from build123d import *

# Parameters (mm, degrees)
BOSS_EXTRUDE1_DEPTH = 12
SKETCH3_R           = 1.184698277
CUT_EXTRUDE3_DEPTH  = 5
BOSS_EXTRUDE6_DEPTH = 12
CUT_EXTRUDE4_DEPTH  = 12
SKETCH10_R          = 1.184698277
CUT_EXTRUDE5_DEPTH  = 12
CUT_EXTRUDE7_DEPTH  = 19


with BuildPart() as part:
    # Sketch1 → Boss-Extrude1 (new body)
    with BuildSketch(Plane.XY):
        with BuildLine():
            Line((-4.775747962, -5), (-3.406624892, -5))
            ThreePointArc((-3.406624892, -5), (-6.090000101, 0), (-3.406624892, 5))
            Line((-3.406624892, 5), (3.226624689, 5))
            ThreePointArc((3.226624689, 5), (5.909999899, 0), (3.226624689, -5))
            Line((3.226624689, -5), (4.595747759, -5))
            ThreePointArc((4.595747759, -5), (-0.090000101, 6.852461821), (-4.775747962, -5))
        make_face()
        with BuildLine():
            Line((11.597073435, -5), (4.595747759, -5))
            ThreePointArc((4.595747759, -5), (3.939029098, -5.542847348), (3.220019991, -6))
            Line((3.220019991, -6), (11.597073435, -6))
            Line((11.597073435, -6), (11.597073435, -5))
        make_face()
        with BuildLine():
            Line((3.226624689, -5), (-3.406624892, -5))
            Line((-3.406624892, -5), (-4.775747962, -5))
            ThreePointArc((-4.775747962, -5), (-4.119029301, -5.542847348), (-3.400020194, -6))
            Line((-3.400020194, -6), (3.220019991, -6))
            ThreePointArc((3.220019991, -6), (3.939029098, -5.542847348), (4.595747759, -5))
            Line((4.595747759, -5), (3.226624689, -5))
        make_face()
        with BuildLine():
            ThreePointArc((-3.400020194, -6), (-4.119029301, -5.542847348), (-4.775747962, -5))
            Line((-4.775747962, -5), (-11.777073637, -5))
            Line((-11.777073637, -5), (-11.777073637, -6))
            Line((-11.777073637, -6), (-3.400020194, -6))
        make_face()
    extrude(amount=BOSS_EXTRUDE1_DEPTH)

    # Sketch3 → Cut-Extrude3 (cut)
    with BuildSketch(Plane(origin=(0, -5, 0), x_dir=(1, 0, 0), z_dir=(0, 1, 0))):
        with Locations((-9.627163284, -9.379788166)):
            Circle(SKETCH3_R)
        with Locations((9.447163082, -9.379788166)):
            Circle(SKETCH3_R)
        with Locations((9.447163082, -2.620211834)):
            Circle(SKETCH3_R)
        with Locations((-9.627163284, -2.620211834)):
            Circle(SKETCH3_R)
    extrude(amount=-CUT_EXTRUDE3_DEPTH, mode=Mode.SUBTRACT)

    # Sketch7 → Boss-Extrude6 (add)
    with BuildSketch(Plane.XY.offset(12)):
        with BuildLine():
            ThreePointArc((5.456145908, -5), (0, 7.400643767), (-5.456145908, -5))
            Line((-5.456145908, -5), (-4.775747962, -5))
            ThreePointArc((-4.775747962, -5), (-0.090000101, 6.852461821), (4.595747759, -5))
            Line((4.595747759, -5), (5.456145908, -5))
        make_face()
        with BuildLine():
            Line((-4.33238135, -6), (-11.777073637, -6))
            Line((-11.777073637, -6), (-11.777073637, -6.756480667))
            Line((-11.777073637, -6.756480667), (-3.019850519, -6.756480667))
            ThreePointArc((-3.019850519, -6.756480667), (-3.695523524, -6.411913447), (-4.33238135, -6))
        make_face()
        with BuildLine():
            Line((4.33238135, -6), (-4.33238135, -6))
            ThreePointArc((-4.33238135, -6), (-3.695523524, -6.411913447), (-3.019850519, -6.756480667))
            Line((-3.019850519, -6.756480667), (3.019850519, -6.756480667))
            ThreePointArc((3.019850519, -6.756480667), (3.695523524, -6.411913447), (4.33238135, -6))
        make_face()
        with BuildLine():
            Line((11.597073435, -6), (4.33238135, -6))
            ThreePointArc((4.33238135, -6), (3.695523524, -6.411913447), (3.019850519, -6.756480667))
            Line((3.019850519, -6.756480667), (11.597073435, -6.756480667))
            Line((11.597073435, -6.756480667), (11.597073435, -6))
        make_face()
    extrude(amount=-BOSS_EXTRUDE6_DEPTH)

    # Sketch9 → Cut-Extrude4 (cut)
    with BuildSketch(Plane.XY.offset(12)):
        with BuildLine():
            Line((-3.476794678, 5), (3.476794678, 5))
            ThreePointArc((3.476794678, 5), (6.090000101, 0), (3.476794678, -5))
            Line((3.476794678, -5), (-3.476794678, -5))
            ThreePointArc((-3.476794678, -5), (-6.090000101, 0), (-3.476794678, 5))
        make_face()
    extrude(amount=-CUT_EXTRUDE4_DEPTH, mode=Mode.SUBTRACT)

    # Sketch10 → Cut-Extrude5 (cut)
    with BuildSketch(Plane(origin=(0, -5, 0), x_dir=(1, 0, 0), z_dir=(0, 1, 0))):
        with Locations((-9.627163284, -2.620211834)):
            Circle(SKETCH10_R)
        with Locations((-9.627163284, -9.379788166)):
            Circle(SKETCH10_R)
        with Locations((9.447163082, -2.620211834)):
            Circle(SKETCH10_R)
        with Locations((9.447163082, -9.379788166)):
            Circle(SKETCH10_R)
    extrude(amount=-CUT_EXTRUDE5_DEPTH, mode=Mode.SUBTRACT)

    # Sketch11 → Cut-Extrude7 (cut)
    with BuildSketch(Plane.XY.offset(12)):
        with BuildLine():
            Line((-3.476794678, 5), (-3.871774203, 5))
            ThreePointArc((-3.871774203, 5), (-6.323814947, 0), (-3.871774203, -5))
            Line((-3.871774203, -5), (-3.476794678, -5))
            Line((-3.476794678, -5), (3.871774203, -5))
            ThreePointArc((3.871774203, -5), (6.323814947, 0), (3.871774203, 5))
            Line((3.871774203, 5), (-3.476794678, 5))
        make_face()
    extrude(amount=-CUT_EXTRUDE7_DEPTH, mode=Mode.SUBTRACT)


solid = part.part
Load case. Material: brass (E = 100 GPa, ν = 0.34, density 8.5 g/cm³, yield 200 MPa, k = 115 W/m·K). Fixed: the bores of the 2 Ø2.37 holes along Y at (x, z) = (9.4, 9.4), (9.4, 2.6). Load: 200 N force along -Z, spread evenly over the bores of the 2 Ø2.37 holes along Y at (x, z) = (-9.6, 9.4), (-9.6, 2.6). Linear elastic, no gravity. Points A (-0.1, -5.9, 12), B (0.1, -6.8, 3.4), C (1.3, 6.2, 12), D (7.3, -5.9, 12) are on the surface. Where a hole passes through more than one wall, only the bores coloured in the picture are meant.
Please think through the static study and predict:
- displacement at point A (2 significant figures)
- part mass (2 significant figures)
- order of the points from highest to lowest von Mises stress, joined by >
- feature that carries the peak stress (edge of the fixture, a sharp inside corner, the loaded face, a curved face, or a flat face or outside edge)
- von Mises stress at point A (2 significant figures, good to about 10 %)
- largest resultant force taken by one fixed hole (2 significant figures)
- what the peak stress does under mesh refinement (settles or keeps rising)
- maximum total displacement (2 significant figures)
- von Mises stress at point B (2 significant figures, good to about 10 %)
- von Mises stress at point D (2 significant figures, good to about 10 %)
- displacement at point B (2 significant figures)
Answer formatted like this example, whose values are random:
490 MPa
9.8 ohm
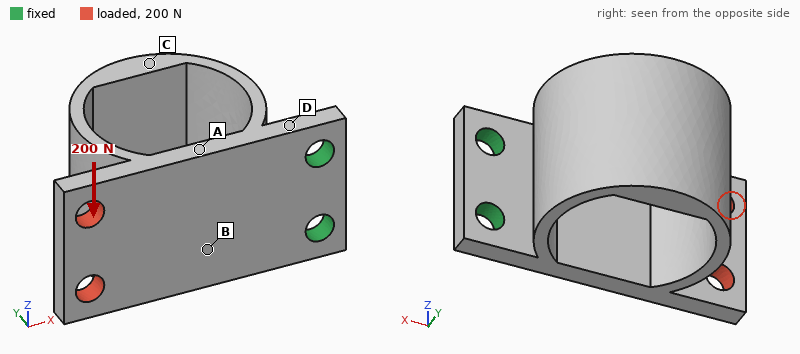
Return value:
11 µm
8.2 g
D > A > B > C
edge of the fixture
45 MPa
470 N
keeps rising
29 µm
29 MPa
60 MPa
8.4 µm
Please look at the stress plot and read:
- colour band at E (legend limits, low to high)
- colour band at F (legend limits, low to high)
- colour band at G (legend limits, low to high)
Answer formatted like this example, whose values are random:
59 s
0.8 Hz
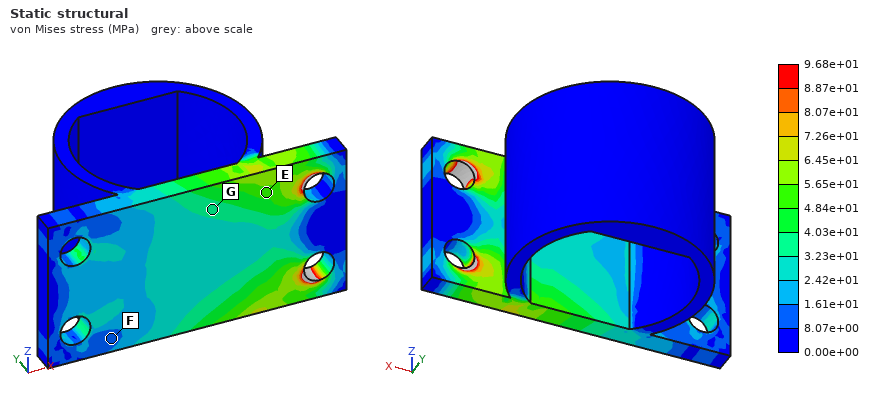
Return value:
4.84e+01 to 5.65e+01 MPa
8.07e+00 to 1.61e+01 MPa
3.23e+01 to 4.03e+01 MPa
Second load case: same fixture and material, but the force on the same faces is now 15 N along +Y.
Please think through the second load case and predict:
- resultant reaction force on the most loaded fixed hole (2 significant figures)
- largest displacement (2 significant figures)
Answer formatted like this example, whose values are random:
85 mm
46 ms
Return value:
7.6 N
54 µm
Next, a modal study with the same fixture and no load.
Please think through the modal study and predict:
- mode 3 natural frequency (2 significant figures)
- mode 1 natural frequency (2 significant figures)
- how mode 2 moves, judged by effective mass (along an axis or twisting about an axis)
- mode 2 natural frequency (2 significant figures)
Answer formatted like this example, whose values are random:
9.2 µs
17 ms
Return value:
5500 Hz
1500 Hz
along Z
4100 Hz
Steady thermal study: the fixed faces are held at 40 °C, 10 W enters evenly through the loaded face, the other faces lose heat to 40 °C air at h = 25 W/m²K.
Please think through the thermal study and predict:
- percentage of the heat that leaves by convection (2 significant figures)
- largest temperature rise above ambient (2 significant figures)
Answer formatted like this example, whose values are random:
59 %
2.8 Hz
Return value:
11 %
70 K
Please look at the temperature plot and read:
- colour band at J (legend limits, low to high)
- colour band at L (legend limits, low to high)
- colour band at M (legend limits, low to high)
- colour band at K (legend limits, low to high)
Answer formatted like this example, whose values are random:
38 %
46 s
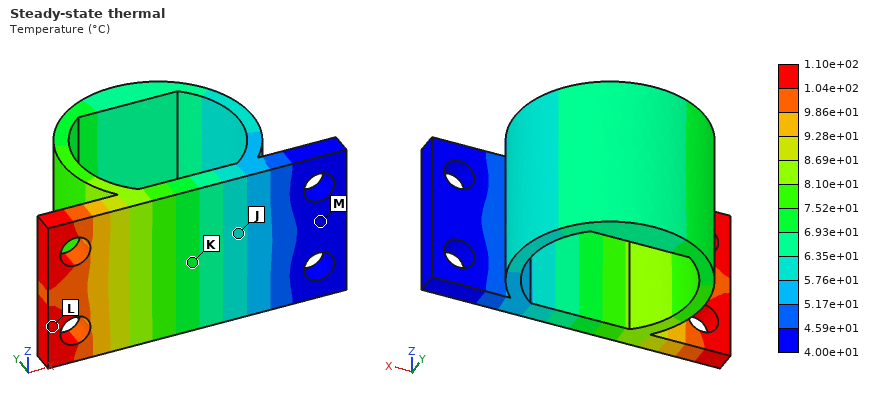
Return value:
5.76e+01 to 6.35e+01 °C
1.04e+02 to 1.10e+02 °C
4.00e+01 to 4.59e+01 °C
6.93e+01 to 7.52e+01 °C
